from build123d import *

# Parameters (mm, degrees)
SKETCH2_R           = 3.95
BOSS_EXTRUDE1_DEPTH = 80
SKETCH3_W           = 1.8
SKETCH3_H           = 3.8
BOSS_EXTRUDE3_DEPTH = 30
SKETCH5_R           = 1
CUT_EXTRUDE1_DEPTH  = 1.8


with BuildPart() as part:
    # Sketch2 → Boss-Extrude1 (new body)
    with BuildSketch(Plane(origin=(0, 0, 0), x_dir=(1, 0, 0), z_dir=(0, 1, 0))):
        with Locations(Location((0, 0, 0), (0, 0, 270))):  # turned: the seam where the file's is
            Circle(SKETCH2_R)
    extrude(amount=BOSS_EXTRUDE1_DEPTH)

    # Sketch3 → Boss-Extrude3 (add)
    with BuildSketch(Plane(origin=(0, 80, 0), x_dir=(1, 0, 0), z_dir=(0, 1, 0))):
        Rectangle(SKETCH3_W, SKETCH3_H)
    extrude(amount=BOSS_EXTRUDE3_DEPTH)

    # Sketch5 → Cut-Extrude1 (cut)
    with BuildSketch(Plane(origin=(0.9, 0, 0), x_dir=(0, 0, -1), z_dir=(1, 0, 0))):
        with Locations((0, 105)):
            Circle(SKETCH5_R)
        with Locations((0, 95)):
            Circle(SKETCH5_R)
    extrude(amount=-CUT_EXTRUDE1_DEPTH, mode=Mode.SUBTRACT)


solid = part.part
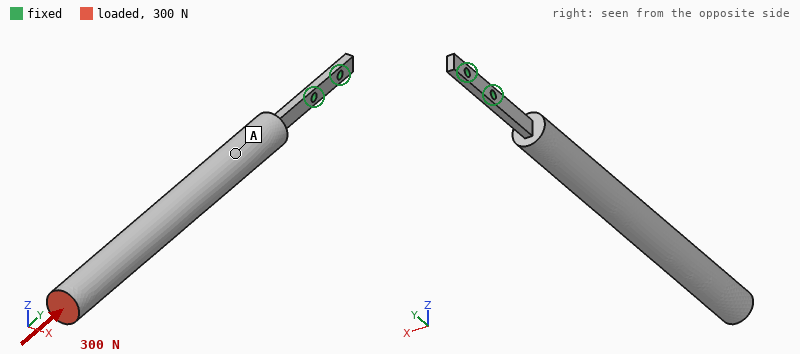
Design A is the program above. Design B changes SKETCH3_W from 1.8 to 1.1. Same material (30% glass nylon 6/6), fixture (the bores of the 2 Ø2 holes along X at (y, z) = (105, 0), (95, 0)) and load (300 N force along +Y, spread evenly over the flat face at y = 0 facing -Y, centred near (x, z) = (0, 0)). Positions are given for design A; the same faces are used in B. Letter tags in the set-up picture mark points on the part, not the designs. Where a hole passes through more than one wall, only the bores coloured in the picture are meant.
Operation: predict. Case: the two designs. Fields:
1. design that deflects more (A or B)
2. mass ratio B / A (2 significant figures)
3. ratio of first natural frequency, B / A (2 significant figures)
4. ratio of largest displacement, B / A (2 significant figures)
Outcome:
B
0.98
0.48
1.4
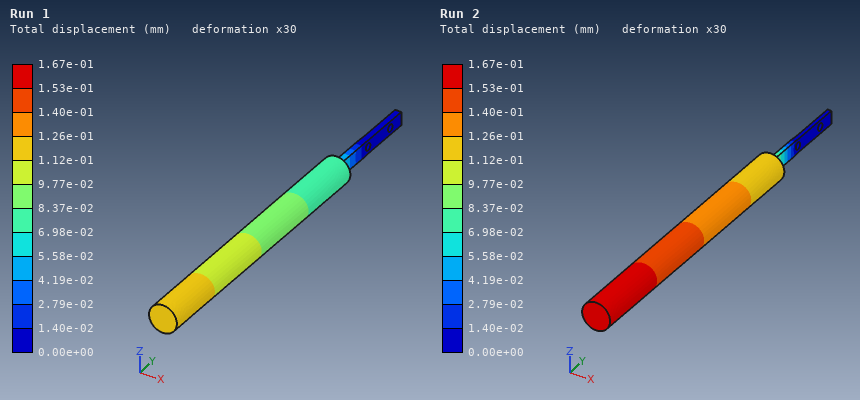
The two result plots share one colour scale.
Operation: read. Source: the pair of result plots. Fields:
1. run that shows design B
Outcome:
Run 2
